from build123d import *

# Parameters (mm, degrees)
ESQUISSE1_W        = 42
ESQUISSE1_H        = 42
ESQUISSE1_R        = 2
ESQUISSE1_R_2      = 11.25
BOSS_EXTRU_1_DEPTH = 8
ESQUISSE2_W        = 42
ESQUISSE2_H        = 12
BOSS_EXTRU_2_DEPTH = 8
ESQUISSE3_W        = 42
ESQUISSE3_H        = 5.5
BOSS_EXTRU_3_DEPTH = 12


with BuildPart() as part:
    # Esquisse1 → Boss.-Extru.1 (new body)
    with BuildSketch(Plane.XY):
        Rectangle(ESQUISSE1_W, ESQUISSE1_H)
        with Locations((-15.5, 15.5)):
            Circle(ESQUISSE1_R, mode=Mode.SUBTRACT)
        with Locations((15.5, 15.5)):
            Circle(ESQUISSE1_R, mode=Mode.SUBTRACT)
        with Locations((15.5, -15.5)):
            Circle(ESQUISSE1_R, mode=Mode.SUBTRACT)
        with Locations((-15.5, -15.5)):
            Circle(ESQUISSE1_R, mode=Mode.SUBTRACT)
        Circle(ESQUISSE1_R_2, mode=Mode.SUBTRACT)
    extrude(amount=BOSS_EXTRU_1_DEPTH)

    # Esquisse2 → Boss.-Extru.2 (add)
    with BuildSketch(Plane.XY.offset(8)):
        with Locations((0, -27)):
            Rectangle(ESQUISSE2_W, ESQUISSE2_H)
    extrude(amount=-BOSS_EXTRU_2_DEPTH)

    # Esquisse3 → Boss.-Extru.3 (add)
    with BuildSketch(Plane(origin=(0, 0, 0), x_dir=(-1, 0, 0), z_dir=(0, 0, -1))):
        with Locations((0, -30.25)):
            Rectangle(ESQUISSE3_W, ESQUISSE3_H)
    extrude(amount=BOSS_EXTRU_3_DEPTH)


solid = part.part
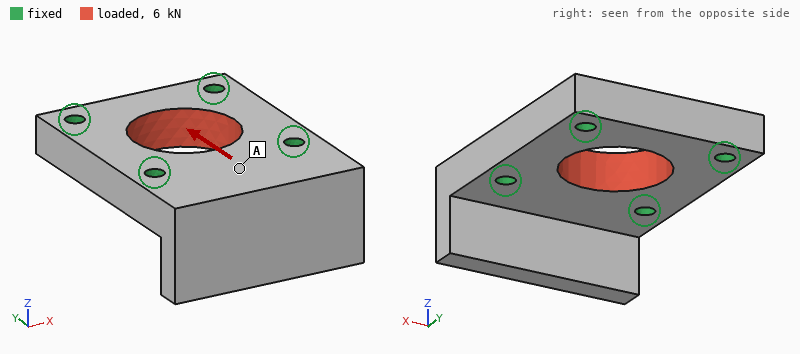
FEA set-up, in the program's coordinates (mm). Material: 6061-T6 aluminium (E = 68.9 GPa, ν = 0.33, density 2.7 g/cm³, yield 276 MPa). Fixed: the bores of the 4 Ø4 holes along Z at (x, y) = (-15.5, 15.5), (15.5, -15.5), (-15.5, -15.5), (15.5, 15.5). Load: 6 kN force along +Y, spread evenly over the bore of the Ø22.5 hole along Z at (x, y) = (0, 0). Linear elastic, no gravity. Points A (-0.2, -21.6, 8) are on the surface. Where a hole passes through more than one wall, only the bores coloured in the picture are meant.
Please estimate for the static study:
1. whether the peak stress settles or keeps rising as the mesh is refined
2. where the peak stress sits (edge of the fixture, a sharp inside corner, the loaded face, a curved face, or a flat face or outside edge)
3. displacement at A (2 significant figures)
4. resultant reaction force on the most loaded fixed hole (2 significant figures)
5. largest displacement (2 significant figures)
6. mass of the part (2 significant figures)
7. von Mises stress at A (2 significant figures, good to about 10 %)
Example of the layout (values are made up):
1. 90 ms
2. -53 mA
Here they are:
1. keeps rising
2. edge of the fixture
3. 2.5 µm
4. 1.6 kN
5. 7.2 µm
6. 47 g
7. 6.0 MPa
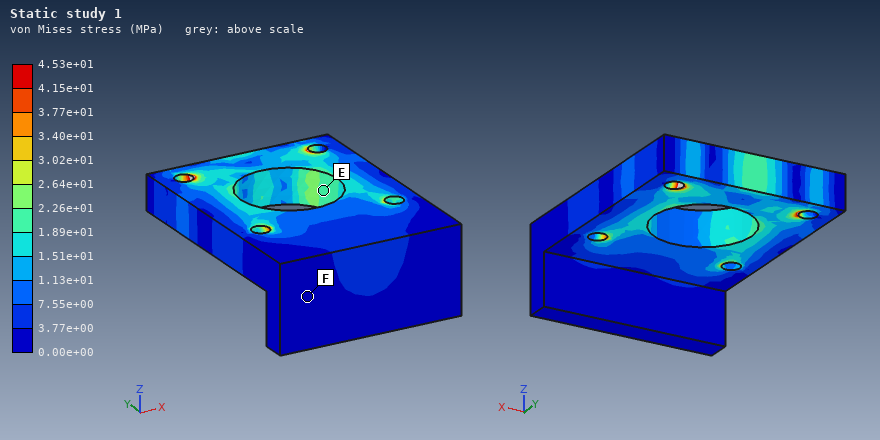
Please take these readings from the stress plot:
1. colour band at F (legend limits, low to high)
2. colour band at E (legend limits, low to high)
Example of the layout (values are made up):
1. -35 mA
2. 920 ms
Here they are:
1. 0.00e+00 to 3.77e+00 MPa
2. 1.89e+01 to 2.26e+01 MPa
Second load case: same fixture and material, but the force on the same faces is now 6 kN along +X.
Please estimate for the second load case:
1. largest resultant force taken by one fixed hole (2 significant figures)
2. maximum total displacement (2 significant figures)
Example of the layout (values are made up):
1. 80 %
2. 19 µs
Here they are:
1. 1.6 kN
2. 6.6 µm
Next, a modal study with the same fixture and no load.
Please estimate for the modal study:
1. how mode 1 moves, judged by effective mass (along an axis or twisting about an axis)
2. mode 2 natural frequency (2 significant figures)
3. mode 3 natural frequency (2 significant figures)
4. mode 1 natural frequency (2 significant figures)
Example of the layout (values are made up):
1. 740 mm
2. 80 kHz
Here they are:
1. along Z
2. 14 kHz
3. 20 kHz
4. 9000 Hz
